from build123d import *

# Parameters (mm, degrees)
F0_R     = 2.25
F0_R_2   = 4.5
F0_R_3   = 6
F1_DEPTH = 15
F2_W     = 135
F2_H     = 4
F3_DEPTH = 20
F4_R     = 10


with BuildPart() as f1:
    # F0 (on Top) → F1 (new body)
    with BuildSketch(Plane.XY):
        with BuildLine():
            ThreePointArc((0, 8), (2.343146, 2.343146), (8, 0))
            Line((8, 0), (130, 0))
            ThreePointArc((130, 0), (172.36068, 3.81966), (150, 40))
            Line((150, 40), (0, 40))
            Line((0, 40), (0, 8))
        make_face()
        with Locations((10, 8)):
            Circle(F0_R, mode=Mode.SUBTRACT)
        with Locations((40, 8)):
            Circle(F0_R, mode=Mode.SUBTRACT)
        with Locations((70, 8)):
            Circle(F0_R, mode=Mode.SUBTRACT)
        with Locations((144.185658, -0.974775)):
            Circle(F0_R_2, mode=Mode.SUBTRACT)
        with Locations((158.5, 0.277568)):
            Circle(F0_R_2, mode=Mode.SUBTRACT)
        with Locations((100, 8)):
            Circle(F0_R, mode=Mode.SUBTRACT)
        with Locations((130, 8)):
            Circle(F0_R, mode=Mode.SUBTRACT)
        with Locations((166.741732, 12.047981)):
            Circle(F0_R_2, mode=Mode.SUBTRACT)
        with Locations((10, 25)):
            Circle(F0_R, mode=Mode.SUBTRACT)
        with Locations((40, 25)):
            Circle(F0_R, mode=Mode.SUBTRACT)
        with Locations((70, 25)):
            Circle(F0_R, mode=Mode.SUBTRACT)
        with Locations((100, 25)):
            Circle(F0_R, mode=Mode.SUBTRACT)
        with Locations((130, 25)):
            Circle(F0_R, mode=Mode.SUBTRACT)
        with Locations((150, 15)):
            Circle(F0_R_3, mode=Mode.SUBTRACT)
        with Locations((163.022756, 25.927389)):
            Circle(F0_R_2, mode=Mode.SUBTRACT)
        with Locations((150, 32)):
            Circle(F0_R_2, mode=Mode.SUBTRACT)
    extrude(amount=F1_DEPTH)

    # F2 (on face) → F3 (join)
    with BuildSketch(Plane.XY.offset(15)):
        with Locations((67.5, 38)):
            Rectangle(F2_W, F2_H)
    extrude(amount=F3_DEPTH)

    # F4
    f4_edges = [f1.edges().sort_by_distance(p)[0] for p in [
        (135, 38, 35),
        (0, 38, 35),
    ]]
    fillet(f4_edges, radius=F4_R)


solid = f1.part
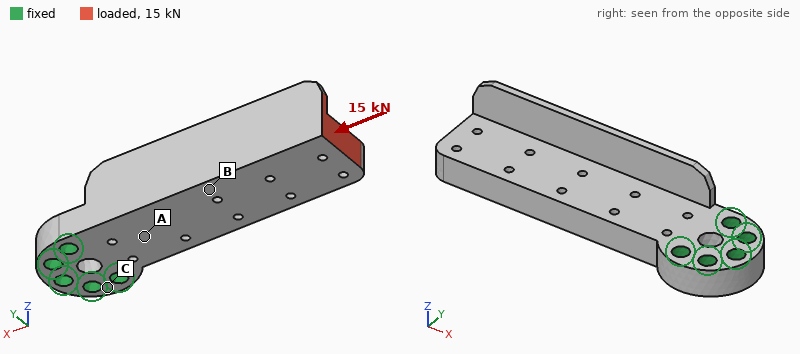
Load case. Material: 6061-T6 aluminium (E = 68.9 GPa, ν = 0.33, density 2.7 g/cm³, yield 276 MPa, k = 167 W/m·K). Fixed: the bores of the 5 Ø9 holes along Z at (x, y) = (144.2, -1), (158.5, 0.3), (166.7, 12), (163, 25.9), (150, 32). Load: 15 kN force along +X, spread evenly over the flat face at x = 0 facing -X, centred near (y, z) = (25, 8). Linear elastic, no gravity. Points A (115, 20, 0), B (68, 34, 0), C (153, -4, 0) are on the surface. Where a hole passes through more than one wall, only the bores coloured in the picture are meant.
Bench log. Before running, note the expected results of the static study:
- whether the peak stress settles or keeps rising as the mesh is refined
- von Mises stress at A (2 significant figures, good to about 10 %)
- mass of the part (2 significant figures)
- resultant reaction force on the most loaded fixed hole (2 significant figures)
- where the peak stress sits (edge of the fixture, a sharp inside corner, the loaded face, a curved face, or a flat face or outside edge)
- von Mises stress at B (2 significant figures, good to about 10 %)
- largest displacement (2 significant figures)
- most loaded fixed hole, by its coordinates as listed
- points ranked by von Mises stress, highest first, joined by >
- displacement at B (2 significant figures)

keeps rising
24 MPa
290 g
11 kN
edge of the fixture
39 MPa
0.15 mm
(150, 32)
B > A > C
0.064 mm
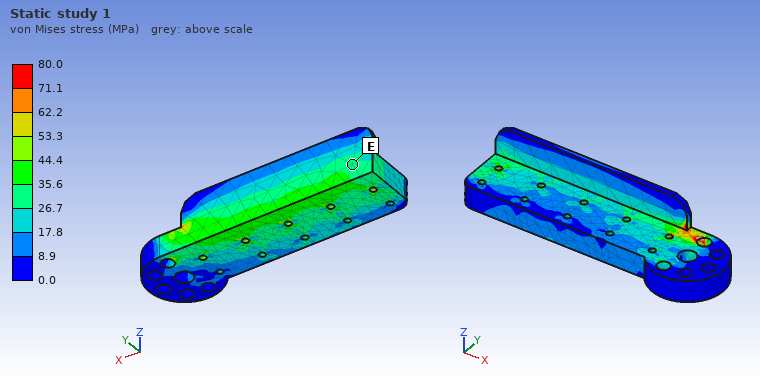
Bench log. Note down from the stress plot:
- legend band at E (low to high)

26.7 to 35.6 MPa
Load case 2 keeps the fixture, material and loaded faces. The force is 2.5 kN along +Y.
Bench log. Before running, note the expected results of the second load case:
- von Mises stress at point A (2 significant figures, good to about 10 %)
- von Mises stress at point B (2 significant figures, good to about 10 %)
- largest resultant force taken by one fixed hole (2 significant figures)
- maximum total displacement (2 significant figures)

14 MPa
35 MPa
10 kN
0.50 mm
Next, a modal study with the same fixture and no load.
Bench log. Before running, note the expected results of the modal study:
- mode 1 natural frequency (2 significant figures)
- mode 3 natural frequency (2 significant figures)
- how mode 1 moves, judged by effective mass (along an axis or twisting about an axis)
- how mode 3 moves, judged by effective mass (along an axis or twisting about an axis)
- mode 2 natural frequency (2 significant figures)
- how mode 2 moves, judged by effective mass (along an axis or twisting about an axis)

610 Hz
2800 Hz
along Z
twisting about X
1500 Hz
along Y
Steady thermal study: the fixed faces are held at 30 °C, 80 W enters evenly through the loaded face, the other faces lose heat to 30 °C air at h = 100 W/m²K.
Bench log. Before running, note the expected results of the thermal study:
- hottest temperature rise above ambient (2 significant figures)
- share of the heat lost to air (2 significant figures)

61 K
68 %
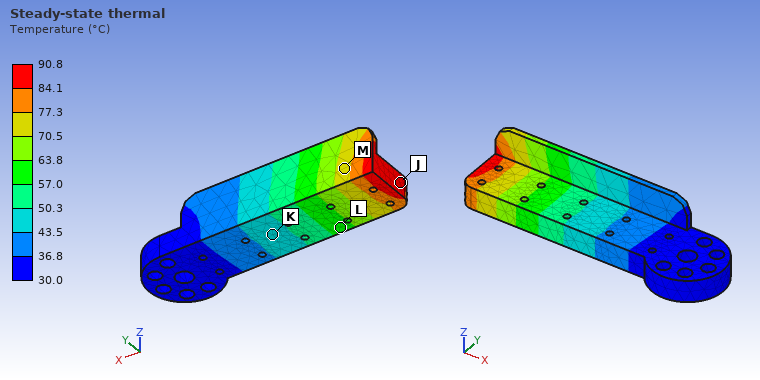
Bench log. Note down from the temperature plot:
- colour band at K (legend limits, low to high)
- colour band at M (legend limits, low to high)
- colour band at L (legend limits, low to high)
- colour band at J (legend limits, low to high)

43.5 to 50.3 °C
70.5 to 77.3 °C
57.0 to 63.8 °C
84.1 to 90.8 °C
